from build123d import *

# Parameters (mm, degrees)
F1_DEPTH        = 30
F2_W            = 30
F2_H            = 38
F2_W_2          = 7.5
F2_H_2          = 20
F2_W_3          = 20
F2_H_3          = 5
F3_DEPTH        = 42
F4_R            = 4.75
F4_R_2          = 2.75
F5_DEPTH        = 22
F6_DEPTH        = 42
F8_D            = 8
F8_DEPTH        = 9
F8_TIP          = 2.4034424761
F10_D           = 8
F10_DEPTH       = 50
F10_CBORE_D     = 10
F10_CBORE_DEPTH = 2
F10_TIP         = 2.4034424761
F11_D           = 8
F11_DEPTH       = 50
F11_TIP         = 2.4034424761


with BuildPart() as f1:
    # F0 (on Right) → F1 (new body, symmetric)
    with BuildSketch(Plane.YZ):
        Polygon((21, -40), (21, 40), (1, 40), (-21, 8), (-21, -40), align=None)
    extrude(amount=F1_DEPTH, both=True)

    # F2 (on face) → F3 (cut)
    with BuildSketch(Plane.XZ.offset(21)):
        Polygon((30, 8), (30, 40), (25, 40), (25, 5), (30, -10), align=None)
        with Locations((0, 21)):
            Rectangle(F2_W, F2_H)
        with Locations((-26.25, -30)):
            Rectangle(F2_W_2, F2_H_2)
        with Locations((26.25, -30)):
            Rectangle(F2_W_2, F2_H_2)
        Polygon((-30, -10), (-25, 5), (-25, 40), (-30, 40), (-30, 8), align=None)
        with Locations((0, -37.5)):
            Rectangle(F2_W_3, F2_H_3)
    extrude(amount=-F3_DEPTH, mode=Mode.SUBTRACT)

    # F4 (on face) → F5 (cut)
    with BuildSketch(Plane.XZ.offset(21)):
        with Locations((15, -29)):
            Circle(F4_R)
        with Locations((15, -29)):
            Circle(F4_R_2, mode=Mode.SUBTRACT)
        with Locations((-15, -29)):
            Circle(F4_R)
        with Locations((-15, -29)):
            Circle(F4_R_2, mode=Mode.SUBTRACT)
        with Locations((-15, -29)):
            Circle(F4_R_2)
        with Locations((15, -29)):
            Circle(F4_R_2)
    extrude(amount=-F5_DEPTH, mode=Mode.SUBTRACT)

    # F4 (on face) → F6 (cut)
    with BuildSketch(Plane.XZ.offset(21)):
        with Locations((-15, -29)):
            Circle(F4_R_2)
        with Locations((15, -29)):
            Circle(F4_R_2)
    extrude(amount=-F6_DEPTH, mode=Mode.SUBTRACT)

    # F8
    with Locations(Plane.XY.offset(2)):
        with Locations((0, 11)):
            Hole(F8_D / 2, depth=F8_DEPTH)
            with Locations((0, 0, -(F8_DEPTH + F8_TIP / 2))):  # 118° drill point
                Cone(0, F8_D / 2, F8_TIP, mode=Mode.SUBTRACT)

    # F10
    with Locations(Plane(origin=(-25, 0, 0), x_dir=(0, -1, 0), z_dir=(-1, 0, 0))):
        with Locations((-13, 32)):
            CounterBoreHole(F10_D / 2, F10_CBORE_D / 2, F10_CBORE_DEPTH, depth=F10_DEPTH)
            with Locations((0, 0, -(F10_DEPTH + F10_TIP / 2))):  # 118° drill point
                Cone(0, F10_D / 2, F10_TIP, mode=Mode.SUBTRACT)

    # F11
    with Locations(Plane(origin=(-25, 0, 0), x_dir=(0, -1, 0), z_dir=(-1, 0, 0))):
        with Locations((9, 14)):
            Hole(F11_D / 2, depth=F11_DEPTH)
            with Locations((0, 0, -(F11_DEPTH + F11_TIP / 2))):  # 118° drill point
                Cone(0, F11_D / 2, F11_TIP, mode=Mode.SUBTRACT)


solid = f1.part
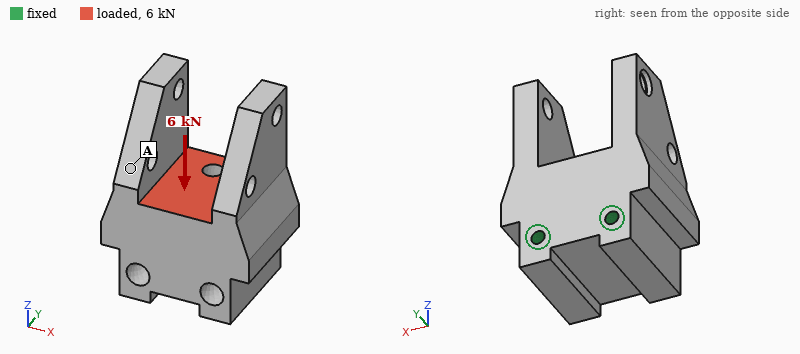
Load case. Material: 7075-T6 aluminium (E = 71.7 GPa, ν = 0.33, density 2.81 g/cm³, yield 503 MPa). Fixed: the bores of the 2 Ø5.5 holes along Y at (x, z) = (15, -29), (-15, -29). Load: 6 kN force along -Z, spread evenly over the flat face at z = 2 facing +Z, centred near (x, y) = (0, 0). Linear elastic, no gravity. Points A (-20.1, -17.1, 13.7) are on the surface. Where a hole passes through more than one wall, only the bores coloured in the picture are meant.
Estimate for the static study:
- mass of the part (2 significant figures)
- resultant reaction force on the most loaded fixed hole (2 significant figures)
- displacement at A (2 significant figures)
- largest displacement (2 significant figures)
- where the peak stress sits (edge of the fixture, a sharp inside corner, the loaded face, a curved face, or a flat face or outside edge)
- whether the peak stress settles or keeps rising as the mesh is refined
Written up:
300 g
3.1 kN
16 µm
21 µm
edge of the fixture
keeps rising
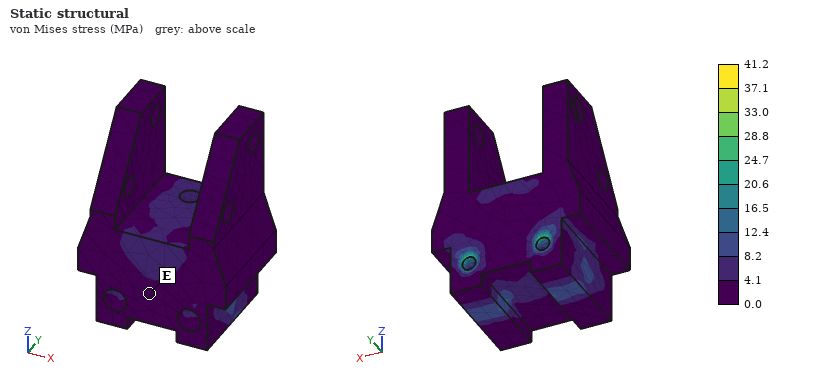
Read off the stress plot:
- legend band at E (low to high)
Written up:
0.0 to 4.1 MPa
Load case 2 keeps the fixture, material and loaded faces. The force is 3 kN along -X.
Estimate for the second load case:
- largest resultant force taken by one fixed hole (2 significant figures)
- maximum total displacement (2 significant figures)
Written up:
3.3 kN
12 µm
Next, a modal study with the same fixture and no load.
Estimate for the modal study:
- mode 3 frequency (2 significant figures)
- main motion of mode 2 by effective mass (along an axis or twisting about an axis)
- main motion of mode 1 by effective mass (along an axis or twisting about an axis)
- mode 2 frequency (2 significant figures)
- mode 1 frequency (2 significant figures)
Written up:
5400 Hz
along X
along Y
4800 Hz
4300 Hz
